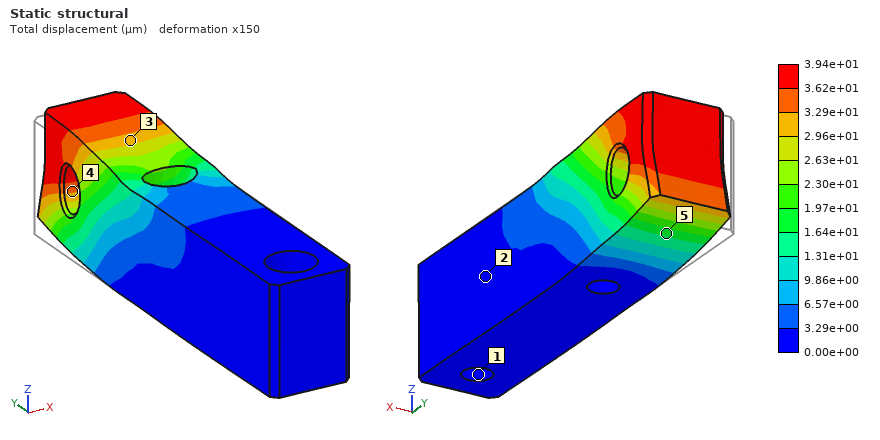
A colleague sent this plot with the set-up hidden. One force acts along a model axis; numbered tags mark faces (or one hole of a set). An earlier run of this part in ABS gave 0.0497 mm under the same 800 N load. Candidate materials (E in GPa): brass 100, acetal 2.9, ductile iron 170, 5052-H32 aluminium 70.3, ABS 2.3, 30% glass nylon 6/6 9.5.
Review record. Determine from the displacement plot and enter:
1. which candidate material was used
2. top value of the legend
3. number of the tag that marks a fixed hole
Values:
acetal
3.94e+01 µm
1
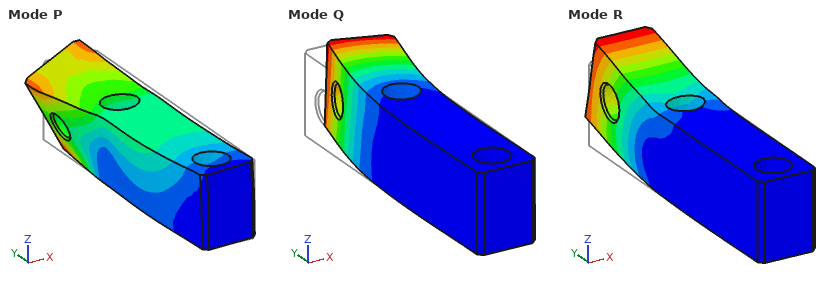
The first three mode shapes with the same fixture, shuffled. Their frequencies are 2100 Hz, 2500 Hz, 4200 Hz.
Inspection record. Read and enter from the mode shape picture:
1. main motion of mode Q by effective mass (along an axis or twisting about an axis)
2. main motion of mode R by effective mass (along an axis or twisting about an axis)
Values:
along X
along Z
